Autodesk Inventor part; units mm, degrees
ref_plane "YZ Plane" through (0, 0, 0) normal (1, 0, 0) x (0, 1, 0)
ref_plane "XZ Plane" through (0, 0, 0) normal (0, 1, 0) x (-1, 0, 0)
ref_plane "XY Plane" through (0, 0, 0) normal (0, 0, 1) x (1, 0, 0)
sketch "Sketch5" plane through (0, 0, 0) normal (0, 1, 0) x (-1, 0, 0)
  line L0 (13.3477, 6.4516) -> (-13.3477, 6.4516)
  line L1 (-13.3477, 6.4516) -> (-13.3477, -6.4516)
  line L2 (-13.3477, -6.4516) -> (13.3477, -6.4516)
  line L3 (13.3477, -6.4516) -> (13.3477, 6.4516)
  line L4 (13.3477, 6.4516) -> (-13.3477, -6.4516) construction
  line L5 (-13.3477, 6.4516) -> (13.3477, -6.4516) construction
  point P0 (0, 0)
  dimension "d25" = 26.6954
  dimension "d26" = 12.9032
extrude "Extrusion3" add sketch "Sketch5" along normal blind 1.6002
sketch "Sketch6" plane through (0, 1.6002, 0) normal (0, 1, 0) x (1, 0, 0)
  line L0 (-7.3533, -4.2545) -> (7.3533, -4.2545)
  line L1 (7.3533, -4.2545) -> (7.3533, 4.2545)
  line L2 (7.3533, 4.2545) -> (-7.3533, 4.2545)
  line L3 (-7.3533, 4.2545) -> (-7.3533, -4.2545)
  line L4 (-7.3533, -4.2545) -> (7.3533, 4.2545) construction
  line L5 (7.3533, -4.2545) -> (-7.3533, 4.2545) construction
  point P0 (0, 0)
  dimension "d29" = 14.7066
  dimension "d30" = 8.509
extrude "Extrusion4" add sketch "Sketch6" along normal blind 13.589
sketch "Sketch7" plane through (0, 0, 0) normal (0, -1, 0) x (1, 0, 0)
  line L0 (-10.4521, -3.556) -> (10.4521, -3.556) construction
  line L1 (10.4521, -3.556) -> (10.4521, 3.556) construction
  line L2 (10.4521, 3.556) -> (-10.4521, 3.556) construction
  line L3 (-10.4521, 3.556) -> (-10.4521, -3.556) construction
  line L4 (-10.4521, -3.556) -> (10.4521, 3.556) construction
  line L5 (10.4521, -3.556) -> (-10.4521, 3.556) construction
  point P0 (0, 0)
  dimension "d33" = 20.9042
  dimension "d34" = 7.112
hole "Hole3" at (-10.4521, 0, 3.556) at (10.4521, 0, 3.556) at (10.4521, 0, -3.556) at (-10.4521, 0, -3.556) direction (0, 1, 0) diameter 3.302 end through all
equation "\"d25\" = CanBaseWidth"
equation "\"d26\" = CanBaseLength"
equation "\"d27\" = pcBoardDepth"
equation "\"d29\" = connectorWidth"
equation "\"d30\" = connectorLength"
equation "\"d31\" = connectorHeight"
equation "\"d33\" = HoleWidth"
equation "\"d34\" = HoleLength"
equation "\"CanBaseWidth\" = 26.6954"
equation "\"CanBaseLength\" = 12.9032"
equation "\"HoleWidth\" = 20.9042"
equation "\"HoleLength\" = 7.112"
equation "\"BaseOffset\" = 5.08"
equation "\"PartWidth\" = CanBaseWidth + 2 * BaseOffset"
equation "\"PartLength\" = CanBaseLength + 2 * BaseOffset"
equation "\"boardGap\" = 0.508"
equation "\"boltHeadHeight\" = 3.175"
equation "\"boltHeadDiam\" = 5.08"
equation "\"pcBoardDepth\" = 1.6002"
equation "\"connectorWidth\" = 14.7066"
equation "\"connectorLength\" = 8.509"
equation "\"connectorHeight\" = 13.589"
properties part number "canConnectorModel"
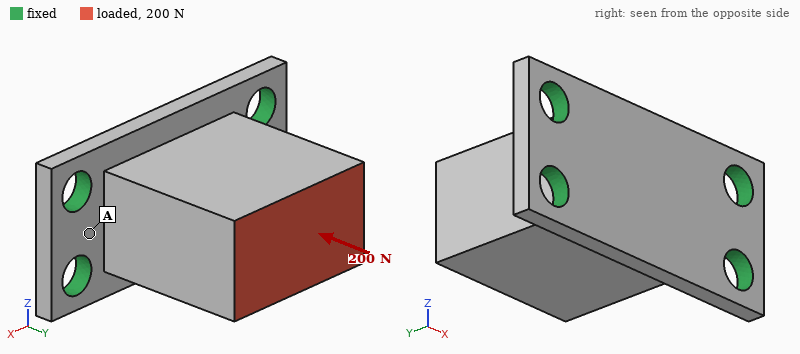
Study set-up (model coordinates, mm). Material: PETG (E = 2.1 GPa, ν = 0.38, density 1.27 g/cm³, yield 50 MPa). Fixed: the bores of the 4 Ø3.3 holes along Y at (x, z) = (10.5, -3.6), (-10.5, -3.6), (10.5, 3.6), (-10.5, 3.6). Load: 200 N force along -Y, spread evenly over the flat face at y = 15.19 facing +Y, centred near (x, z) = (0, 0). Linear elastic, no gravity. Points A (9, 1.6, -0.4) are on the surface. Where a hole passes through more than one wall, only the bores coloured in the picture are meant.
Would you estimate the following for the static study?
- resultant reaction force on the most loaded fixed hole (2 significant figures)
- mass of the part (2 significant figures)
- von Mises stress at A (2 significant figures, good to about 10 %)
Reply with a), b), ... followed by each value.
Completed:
a) 57 N
b) 2.8 g
c) 4.9 MPa
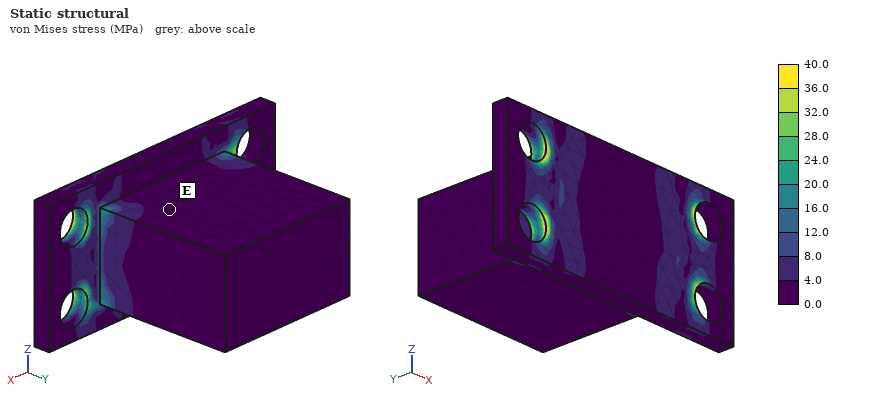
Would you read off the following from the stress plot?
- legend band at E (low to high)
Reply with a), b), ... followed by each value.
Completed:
a) 0.0 to 4.0 MPa
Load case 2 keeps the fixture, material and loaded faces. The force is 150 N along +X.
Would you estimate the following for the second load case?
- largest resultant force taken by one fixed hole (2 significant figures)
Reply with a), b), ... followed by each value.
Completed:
a) 78 N
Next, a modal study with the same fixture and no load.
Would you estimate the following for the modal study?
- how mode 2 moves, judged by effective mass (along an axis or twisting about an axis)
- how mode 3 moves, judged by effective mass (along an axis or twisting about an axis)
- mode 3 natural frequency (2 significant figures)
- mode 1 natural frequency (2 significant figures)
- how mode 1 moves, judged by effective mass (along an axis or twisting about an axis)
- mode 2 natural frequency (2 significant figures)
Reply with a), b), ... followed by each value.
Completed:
a) along X
b) along Y
c) 6100 Hz
d) 2500 Hz
e) along Z
f) 5300 Hz
